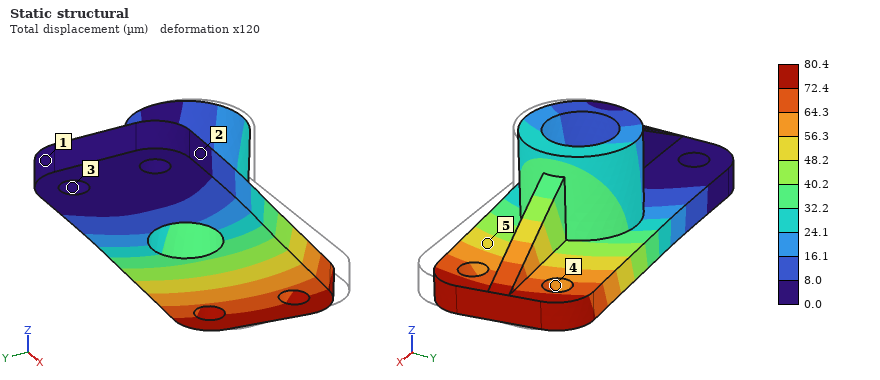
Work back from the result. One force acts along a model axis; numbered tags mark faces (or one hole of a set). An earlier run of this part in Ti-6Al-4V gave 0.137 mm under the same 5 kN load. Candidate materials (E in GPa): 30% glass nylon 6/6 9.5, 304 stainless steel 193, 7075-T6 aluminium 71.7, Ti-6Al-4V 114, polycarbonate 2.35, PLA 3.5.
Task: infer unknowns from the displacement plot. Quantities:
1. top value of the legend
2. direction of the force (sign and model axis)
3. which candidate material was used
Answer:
80.4 µm
+Y
304 stainless steel
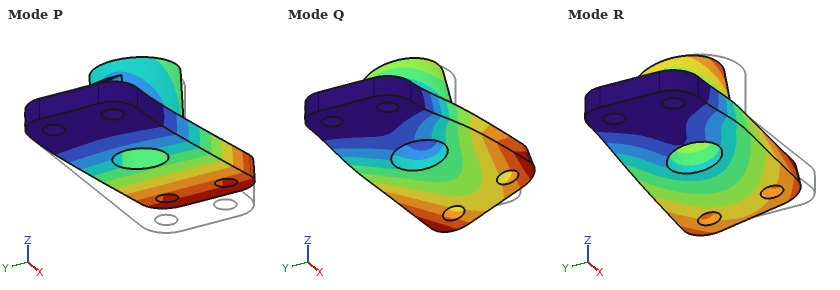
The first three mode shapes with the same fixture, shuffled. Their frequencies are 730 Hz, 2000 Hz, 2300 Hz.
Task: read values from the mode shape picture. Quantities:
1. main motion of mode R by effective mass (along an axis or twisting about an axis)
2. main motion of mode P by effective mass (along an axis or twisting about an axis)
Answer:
along Y
along Z
